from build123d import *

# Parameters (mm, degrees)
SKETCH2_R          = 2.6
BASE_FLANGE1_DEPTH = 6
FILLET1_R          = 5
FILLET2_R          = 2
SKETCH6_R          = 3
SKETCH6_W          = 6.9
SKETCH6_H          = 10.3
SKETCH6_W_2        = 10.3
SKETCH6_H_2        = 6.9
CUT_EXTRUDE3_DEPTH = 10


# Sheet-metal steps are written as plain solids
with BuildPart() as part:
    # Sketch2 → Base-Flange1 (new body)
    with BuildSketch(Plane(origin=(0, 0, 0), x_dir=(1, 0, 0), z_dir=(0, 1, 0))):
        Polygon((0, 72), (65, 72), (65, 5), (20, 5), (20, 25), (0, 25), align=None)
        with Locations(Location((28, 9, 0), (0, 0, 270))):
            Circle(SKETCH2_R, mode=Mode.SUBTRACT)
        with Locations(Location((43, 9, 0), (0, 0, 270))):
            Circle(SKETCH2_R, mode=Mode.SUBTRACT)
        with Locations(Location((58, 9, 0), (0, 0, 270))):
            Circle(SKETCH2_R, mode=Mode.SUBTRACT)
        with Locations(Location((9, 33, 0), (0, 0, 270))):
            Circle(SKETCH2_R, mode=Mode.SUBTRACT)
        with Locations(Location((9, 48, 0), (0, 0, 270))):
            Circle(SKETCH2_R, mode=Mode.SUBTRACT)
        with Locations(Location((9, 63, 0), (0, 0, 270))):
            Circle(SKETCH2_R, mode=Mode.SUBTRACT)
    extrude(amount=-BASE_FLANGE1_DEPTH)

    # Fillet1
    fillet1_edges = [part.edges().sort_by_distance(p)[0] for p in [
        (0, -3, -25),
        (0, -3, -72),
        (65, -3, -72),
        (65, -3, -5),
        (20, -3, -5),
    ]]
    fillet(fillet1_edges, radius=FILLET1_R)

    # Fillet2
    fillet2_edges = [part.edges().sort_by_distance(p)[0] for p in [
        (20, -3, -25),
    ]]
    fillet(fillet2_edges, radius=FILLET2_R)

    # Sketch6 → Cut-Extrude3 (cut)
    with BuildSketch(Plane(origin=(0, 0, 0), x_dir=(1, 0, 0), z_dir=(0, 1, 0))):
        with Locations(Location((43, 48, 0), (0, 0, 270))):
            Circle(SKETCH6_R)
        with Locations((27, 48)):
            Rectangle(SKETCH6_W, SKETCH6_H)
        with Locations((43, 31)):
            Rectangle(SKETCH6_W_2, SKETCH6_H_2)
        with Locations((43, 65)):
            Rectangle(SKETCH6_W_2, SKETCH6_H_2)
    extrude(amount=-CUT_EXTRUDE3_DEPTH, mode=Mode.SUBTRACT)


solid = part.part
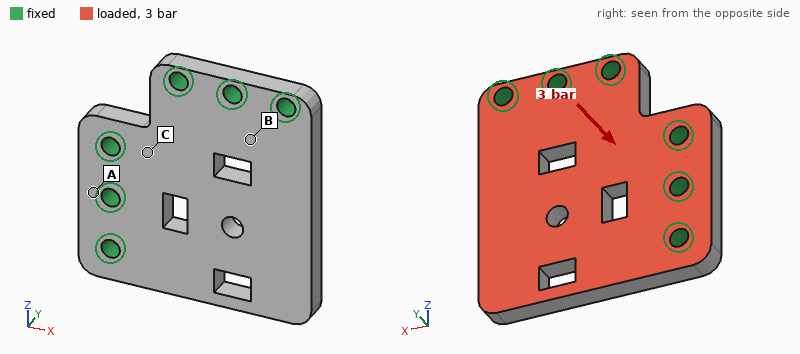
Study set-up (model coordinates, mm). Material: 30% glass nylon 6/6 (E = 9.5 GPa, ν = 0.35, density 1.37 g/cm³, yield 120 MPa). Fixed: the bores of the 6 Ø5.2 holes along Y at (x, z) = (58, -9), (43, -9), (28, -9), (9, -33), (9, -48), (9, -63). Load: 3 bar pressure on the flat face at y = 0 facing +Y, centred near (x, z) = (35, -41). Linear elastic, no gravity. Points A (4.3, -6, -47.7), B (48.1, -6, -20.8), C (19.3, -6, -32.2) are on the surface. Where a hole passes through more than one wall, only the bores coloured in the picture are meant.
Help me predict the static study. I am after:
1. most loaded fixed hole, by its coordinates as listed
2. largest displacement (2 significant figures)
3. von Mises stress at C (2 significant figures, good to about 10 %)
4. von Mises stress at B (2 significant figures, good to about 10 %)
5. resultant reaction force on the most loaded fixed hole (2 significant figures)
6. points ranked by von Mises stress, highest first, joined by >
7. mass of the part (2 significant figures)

(9, -63)
0.87 mm
9.6 MPa
16 MPa
300 N
B > C > A
29 g
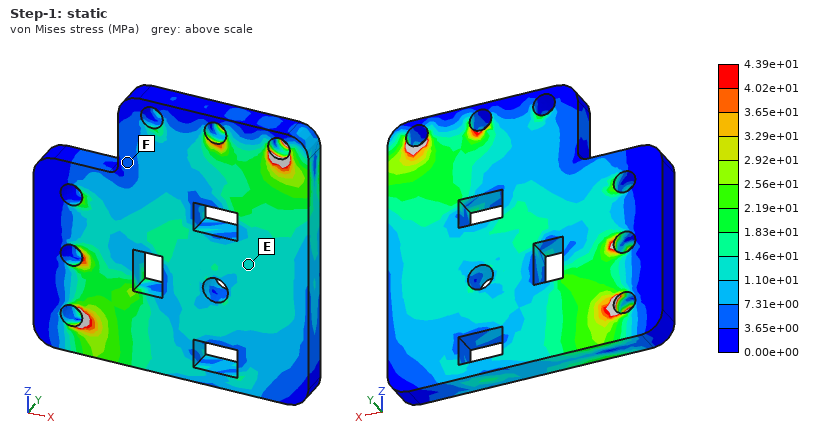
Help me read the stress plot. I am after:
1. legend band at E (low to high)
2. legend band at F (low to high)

1.10e+01 to 1.46e+01 MPa
3.65e+00 to 7.31e+00 MPa
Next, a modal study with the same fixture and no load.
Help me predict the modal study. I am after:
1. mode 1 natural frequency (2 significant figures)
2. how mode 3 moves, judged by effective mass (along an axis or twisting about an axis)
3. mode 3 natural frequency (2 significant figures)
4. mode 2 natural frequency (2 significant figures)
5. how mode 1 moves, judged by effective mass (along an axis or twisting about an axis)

1400 Hz
along Y
5400 Hz
4600 Hz
along Y
